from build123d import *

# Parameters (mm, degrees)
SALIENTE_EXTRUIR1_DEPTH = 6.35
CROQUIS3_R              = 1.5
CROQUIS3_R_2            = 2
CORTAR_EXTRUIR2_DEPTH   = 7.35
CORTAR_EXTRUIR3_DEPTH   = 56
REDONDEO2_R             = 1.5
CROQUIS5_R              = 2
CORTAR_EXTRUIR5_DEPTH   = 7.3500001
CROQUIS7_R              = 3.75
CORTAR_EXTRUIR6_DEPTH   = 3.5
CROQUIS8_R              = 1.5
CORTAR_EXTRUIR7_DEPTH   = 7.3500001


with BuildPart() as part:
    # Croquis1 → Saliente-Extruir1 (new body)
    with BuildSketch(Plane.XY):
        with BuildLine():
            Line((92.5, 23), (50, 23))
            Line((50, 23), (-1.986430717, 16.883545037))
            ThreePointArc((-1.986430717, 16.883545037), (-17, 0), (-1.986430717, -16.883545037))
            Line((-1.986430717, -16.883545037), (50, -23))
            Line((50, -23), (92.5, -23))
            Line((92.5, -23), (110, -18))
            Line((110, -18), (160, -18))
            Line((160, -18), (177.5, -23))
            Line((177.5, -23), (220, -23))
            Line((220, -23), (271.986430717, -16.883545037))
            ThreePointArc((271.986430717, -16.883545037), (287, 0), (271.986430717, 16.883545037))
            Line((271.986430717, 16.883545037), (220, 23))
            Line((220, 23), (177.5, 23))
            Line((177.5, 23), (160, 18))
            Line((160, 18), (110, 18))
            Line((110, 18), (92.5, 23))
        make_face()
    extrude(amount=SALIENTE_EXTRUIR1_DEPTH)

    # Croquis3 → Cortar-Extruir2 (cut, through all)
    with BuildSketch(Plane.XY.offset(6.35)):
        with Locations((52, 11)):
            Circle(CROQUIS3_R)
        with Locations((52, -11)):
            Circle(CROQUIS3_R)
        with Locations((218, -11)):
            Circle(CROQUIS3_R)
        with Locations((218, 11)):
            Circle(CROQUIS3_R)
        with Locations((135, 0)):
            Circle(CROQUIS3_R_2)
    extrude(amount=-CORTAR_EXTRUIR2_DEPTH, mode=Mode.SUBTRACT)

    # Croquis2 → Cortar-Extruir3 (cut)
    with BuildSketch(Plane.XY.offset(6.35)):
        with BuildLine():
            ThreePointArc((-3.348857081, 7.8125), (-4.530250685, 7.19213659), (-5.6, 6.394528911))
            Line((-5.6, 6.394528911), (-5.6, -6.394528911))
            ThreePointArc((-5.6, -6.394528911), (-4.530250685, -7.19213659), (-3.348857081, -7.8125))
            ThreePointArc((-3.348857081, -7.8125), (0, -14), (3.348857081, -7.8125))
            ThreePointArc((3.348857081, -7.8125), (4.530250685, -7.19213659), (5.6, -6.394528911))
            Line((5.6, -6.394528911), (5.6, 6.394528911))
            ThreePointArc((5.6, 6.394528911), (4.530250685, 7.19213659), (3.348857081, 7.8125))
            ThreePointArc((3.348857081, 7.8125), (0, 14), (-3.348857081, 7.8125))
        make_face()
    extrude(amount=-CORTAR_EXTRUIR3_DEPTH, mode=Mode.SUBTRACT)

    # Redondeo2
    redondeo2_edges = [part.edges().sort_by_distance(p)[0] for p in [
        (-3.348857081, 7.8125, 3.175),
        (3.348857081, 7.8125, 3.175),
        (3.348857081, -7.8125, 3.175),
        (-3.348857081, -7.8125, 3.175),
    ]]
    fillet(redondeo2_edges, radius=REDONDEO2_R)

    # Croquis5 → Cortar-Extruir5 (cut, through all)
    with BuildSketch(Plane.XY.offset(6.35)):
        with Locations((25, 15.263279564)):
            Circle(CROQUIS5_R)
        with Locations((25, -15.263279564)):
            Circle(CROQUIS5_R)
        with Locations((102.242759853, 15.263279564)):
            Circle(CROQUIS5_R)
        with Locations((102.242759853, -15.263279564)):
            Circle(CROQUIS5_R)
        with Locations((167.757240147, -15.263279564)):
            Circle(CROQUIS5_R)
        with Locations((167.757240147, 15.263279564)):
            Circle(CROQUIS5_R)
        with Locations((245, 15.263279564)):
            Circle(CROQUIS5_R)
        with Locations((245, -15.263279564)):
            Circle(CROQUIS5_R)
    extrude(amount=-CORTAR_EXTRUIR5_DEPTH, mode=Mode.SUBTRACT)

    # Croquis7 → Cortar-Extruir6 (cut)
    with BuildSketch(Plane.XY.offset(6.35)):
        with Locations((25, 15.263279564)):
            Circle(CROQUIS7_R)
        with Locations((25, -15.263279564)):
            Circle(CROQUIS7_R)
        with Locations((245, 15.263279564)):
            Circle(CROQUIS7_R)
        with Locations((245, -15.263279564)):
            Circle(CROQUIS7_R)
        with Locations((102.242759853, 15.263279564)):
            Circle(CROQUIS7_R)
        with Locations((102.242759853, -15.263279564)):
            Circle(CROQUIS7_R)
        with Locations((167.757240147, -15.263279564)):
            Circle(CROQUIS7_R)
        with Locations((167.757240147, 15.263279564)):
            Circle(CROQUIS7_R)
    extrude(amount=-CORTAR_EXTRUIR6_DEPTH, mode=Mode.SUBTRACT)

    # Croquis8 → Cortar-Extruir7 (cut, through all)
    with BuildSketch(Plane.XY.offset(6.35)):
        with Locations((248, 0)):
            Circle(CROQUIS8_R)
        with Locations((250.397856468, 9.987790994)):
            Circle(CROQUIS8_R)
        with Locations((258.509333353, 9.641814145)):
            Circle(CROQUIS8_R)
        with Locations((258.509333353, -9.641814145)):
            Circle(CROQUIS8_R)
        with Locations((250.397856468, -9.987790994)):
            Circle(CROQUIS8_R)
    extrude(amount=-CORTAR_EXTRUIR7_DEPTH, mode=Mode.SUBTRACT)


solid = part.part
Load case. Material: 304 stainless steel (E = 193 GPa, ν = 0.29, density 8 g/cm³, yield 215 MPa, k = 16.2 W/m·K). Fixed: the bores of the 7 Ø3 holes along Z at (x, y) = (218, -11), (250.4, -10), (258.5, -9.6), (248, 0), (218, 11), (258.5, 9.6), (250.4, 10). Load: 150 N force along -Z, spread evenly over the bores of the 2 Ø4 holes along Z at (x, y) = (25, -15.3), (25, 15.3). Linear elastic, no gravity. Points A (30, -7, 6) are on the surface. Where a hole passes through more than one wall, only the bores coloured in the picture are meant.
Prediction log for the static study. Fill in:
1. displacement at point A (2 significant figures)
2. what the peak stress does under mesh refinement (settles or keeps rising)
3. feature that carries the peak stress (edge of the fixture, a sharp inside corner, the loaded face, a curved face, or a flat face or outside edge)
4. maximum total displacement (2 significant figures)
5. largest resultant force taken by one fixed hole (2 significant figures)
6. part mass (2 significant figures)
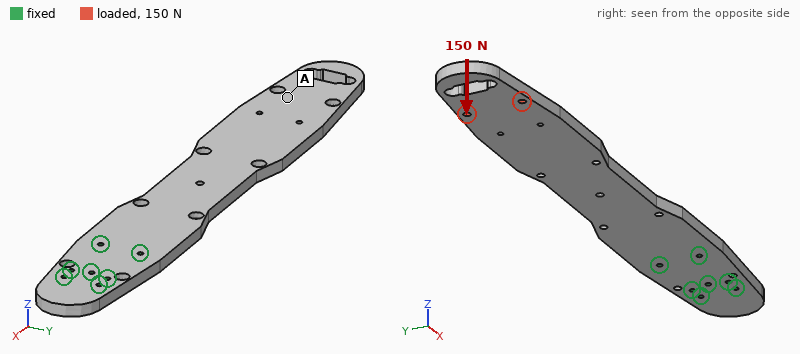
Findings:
2.1 mm
keeps rising
edge of the fixture
3.0 mm
240 N
580 g
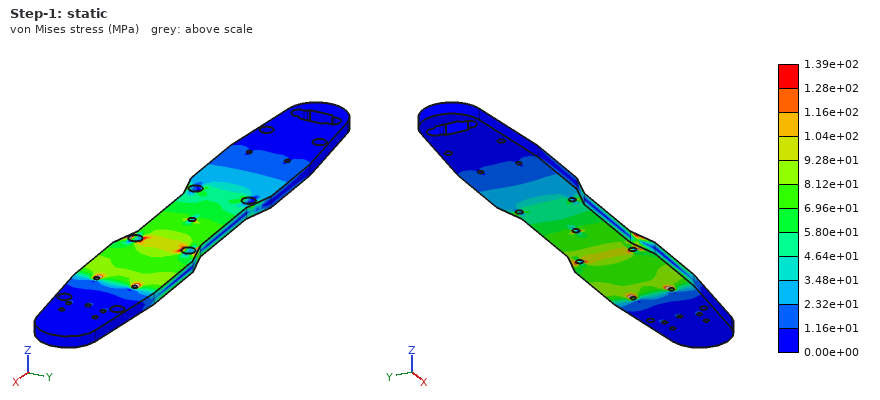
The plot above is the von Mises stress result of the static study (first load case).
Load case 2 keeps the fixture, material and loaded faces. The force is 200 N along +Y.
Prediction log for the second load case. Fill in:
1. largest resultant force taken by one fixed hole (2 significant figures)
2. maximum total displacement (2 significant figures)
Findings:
1.1 kN
0.11 mm
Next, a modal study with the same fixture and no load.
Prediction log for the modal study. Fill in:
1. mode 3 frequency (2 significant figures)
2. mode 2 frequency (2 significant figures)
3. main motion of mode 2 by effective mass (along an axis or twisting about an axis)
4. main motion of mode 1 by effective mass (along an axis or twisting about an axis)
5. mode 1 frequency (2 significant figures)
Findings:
630 Hz
590 Hz
along Y
along Z
100 Hz
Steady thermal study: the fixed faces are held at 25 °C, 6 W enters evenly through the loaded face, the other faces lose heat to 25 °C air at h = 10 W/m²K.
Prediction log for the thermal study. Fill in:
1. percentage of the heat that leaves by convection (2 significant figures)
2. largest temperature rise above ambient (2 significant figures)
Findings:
94 %
75 K
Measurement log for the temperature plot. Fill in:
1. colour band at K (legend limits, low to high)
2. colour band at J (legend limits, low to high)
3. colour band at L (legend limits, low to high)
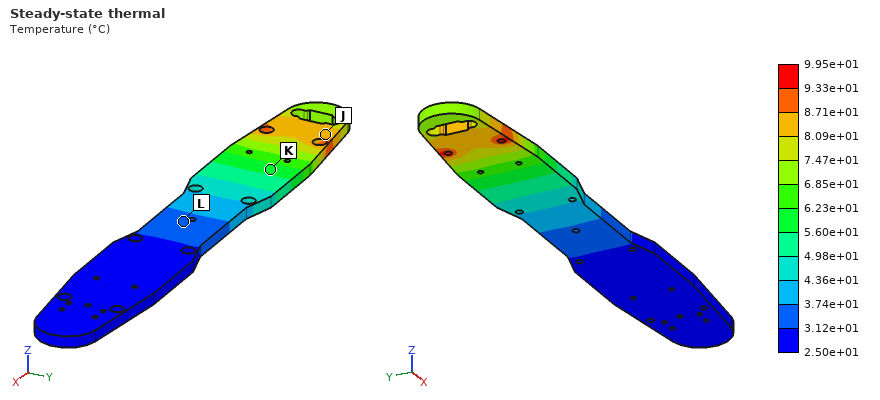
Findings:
5.60e+01 to 6.23e+01 °C
8.09e+01 to 8.71e+01 °C
3.12e+01 to 3.74e+01 °C
